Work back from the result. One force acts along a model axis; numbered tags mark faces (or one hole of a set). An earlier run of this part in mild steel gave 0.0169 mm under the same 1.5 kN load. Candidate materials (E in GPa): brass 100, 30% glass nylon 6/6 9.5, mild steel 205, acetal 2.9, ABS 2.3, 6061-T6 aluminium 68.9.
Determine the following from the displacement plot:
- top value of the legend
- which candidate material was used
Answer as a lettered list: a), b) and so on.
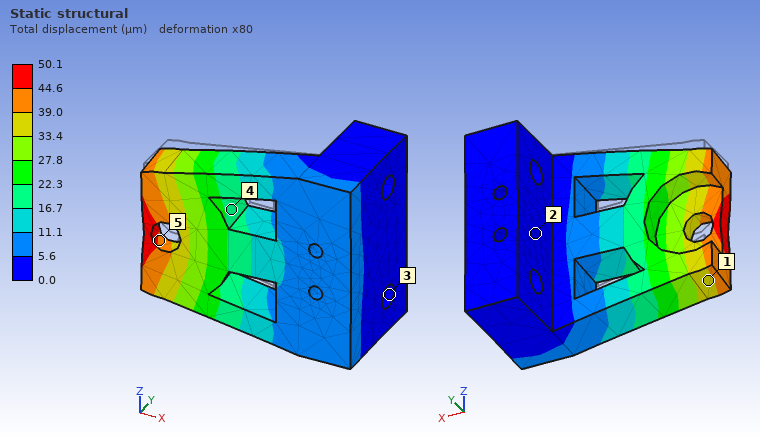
a) 50.1 µm
b) 6061-T6 aluminium
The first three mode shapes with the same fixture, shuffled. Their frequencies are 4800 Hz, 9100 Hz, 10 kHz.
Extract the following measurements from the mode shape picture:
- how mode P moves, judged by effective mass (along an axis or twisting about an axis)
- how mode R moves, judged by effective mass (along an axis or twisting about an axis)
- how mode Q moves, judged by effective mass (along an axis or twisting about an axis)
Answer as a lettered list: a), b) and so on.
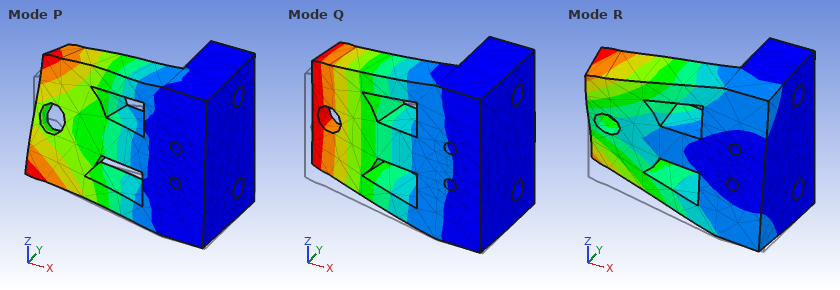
a) along Z
b) along Z
c) along Y
